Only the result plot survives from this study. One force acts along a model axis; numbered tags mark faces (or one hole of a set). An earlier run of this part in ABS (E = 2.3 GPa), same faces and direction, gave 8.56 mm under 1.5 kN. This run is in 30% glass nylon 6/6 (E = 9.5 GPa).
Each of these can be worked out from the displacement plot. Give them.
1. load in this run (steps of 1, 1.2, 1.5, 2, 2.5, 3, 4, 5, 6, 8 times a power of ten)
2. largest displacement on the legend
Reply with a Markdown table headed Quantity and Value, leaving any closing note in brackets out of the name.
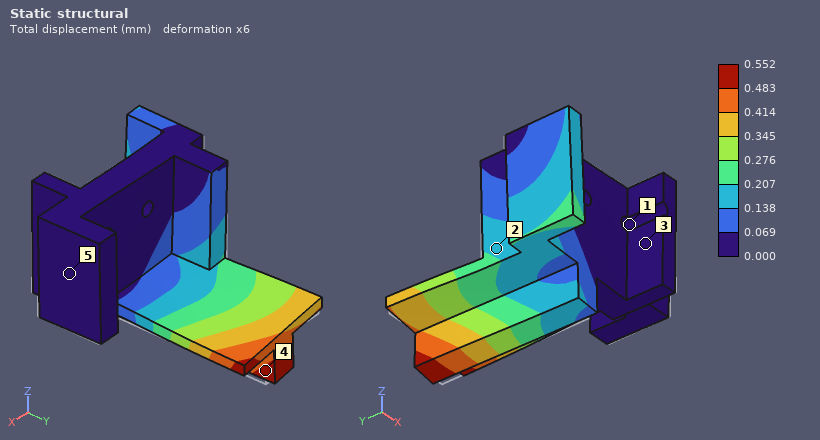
| Quantity | Value |
|---|---|
| load in this run | 400 N |
| largest displacement on the legend | 0.552 mm |
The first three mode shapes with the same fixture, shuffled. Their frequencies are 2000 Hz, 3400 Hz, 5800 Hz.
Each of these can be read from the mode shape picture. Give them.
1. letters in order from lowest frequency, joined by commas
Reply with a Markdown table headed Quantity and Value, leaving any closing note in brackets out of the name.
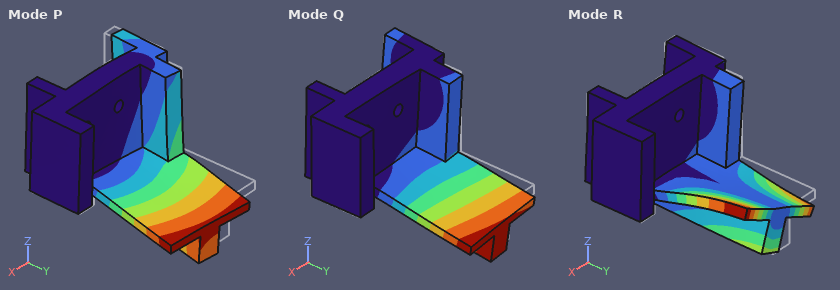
| Quantity | Value |
|---|---|
| letters in order from lowest frequency, joined by commas | Q, P, R |
